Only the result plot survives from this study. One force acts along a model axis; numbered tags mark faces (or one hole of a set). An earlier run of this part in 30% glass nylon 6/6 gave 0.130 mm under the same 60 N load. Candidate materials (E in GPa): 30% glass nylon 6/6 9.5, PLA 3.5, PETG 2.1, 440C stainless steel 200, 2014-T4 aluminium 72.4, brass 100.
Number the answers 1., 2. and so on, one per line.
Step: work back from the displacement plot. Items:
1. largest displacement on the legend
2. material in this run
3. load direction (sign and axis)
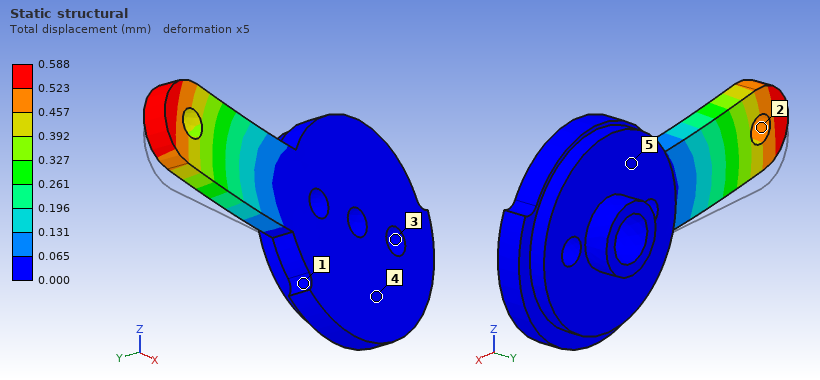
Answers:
1. 0.588 mm
2. PETG
3. +Z
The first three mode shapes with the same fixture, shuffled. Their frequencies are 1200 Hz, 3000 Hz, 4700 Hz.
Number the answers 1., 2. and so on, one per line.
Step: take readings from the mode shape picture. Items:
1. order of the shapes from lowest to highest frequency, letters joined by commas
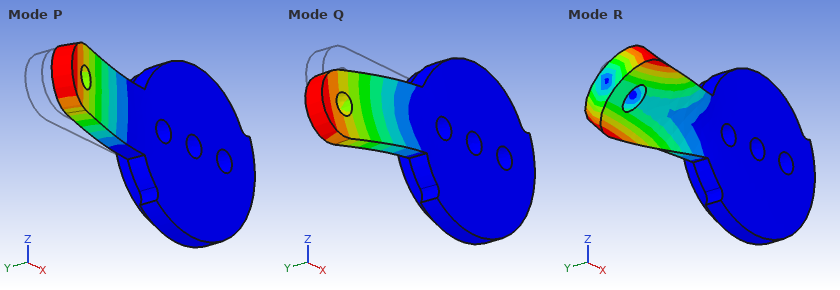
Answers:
1. P, Q, R
